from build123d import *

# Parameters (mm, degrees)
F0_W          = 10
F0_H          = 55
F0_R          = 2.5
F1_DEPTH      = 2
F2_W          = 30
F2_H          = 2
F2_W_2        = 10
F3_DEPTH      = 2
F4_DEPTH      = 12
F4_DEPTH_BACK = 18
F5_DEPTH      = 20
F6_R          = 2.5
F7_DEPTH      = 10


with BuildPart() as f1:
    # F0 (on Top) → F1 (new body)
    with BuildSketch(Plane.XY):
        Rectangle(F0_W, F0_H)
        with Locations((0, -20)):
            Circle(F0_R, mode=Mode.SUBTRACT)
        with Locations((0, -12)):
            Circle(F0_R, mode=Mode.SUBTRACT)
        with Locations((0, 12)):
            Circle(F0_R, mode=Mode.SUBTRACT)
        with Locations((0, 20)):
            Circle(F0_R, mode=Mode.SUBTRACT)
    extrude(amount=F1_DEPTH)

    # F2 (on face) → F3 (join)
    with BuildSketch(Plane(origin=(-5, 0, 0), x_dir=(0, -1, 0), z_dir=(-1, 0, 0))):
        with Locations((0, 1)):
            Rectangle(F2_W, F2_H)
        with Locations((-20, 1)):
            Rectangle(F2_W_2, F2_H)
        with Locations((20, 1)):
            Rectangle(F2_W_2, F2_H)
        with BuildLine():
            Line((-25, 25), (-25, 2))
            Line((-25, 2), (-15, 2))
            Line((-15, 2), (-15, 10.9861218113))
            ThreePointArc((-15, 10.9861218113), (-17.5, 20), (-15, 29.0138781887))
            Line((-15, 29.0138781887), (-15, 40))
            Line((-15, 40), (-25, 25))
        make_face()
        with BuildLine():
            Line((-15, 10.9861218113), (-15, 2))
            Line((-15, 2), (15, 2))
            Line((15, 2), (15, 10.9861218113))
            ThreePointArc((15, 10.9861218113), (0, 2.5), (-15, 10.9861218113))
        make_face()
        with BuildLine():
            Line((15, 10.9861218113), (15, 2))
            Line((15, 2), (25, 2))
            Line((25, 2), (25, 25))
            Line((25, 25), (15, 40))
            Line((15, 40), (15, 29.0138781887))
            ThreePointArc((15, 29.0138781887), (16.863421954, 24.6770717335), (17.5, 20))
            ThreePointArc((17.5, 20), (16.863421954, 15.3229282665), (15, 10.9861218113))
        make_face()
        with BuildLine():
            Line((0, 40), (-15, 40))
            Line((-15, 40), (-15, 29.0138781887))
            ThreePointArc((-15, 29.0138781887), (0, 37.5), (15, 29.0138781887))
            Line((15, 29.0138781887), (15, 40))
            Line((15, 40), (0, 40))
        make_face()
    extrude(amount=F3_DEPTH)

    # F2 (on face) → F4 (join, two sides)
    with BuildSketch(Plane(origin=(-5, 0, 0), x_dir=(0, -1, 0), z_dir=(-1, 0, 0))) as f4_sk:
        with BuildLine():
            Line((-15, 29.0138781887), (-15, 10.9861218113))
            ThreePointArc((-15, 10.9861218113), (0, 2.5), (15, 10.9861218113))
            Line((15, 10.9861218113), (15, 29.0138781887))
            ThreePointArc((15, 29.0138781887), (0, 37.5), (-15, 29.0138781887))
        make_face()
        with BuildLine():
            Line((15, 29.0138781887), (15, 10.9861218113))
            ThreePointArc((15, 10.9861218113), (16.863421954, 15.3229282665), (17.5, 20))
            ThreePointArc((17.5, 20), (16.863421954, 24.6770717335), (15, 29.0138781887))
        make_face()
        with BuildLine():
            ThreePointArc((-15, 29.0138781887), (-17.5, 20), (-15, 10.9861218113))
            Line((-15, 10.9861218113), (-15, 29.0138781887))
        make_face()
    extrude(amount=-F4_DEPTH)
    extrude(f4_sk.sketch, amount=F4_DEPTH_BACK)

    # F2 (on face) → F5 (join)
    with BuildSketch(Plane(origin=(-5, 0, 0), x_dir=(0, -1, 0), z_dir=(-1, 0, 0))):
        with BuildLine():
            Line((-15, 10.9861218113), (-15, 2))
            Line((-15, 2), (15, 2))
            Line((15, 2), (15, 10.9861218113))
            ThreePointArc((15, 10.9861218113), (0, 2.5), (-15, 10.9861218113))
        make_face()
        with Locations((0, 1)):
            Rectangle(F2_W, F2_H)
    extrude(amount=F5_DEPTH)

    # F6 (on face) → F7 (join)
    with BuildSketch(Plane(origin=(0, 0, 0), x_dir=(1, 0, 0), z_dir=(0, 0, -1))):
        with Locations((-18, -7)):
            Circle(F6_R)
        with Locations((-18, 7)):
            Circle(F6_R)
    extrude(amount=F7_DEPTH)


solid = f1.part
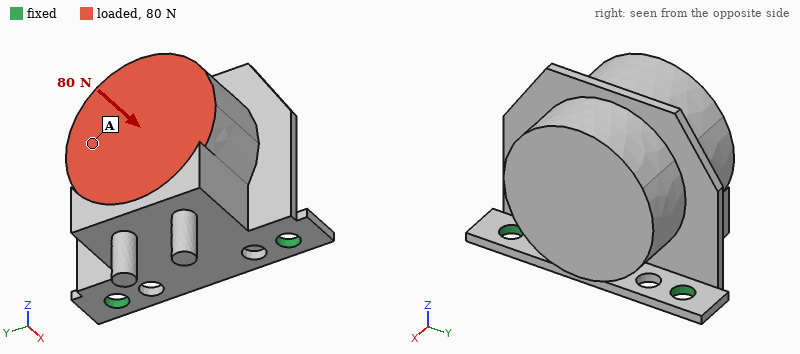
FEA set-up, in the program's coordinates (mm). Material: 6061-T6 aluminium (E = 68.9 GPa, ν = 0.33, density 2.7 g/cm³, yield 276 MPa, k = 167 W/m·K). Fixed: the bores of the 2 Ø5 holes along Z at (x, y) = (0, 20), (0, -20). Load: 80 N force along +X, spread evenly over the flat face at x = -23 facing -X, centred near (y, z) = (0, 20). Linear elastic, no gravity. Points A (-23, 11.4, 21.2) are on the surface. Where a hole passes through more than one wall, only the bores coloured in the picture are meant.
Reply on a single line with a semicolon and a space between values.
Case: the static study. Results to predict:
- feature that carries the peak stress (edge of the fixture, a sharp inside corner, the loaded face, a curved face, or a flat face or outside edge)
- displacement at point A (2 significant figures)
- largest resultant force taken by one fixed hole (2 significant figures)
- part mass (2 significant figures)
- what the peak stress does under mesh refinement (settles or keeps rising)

edge of the fixture; 0.14 mm; 40 N; 94 g; keeps rising
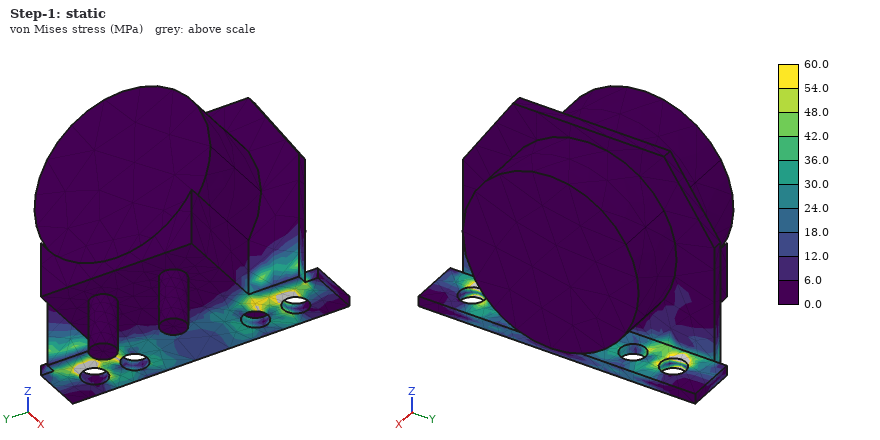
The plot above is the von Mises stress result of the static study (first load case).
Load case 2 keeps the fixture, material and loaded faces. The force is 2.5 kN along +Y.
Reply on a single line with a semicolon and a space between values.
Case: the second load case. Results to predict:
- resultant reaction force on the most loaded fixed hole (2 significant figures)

2.2 kN
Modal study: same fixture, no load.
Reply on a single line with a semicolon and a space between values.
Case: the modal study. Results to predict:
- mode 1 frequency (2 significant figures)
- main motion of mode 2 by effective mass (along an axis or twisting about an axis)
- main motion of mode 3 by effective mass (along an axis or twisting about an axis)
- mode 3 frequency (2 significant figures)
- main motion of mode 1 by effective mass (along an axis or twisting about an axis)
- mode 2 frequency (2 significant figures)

410 Hz; along Y; along Z; 4100 Hz; along X; 3300 Hz
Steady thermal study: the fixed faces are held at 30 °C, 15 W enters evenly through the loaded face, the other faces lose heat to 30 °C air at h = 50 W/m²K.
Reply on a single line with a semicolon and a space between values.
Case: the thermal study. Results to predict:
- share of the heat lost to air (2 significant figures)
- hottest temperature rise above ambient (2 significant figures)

27 %; 13 K
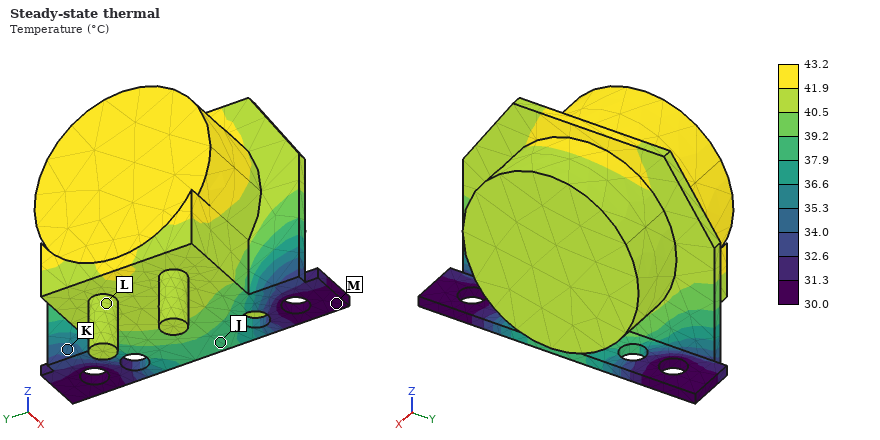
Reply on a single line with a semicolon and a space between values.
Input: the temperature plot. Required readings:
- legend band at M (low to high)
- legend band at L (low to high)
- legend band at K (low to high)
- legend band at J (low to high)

30.0 to 31.3 °C; 40.5 to 41.9 °C; 34.0 to 35.3 °C; 37.9 to 39.2 °C
